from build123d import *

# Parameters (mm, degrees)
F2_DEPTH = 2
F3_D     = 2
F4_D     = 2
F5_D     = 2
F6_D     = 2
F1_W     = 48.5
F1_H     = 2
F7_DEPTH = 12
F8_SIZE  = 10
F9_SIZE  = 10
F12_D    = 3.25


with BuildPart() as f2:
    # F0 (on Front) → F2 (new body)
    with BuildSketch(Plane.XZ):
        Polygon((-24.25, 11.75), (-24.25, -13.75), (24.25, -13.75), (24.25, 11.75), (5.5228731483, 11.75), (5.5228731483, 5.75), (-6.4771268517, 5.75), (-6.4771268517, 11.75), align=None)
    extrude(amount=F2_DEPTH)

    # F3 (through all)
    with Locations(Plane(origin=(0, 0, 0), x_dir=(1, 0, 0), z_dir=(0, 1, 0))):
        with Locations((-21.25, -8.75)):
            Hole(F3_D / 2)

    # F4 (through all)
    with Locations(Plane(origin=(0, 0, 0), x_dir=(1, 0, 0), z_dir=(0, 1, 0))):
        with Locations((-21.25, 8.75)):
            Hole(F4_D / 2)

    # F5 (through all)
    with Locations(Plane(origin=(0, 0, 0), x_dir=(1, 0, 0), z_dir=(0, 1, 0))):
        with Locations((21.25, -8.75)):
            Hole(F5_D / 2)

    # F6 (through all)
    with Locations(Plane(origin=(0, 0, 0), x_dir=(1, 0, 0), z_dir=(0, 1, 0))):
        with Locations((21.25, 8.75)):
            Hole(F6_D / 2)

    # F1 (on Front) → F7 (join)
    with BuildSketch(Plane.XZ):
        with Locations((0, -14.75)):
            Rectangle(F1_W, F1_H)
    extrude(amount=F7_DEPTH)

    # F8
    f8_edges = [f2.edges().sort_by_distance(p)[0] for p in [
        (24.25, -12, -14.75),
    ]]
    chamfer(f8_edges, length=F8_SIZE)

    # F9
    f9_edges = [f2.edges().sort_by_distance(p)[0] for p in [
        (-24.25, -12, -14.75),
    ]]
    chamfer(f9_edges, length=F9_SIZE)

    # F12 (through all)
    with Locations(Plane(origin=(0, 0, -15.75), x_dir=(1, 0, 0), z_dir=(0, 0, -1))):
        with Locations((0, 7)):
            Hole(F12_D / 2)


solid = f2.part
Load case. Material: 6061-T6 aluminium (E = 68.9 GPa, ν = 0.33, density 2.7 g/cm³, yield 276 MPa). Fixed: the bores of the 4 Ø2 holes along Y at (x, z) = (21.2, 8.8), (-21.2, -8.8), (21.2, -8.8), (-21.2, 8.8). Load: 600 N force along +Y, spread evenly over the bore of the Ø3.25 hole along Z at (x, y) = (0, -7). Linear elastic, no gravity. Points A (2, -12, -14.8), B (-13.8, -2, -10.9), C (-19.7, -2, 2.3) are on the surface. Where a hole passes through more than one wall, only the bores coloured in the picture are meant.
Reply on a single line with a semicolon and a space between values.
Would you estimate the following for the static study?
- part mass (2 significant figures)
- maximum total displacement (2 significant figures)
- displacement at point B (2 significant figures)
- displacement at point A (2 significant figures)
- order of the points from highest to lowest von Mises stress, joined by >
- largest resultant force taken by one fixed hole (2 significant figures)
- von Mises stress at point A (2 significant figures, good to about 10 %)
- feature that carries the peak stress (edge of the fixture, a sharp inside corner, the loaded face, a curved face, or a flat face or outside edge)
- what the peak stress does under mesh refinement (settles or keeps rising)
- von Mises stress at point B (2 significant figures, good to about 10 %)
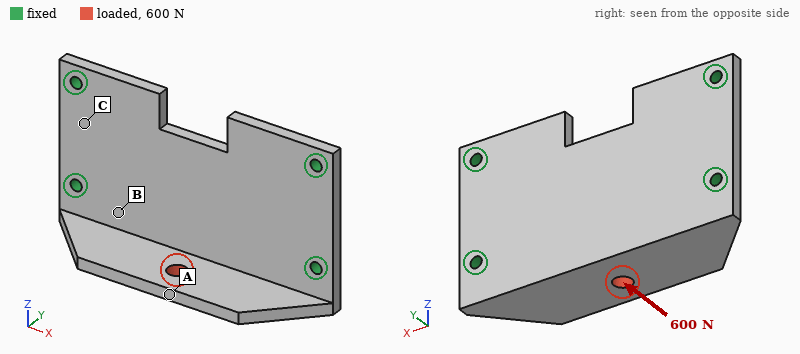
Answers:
8.8 g; 0.12 mm; 0.031 mm; 0.11 mm; A > B > C; 440 N; 97 MPa; edge of the fixture; keeps rising; 53 MPa
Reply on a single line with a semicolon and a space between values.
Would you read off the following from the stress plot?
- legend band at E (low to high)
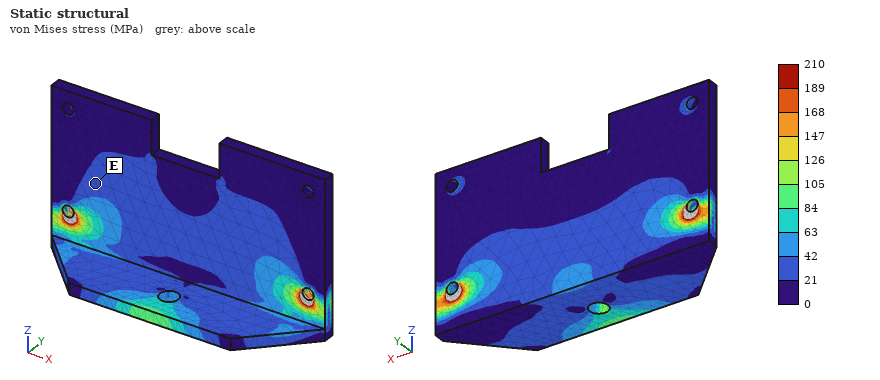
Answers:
21 to 42 MPa
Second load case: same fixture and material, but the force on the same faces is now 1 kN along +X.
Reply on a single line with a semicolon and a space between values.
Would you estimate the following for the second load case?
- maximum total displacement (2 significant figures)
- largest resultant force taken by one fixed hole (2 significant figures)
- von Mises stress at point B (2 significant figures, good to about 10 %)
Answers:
30 µm; 460 N; 39 MPa
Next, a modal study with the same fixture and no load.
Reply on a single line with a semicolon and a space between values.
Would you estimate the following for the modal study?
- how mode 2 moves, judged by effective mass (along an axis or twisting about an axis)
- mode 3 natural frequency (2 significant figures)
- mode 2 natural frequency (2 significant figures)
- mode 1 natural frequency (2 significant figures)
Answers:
along Y; 12 kHz; 7600 Hz; 6200 Hz
